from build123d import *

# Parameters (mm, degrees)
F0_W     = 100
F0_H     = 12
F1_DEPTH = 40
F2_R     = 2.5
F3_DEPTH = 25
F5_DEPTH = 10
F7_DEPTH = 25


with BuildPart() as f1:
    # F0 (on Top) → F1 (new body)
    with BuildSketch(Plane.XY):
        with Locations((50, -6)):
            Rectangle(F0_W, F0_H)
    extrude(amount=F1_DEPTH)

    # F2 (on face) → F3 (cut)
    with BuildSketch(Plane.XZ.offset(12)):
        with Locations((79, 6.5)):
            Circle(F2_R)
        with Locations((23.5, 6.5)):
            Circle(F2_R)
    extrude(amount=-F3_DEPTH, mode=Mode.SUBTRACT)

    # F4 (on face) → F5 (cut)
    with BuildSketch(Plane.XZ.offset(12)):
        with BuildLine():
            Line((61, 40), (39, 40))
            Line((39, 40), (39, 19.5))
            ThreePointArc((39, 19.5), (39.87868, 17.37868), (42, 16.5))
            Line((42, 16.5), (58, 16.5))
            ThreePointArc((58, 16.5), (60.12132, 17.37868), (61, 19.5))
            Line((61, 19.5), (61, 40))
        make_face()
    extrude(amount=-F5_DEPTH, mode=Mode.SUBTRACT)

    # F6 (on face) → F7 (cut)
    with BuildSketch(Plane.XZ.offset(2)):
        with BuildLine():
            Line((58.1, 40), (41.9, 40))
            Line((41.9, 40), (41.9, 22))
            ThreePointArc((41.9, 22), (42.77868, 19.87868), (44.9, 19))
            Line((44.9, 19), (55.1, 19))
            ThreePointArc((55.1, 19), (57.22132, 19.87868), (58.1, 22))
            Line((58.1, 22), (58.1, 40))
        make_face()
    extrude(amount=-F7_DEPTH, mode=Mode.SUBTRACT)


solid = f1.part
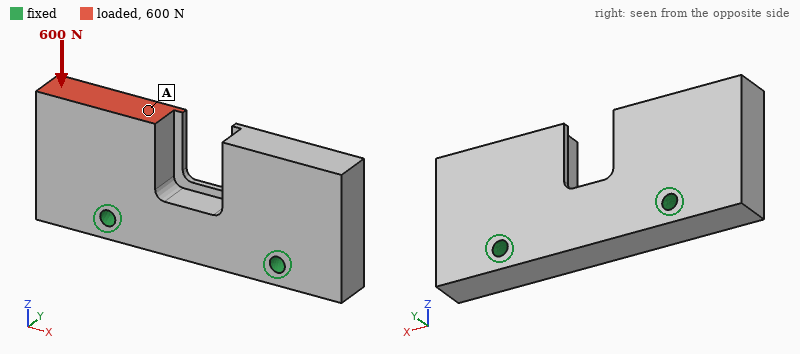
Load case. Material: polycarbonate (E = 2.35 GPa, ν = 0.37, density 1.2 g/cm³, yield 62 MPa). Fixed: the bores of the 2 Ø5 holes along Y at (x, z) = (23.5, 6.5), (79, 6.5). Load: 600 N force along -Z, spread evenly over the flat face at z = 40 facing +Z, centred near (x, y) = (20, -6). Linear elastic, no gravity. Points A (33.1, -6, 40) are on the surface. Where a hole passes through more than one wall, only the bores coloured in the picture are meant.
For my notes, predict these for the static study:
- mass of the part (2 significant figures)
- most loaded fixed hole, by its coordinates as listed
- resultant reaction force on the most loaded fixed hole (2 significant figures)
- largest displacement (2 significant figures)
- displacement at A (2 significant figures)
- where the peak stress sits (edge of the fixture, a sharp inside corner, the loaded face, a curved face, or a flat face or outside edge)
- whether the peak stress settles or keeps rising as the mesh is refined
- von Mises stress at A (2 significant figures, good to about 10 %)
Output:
50 g
(23.5, 6.5)
620 N
97 µm
55 µm
edge of the fixture
keeps rising
1.3 MPa
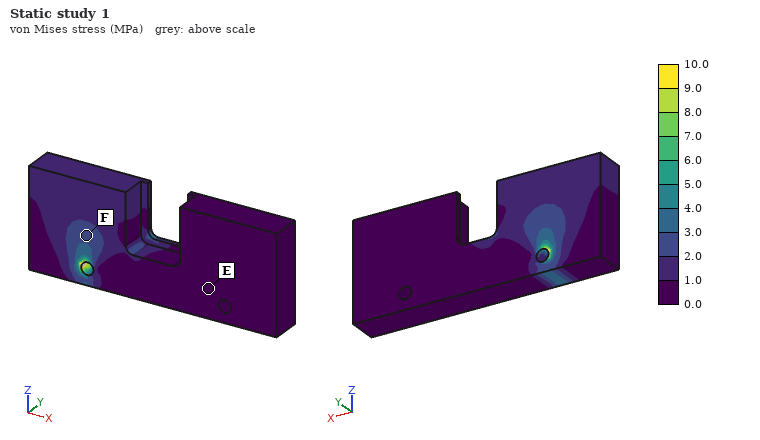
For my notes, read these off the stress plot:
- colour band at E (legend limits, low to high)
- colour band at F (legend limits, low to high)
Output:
0.0 to 1.0 MPa
2.0 to 3.0 MPa
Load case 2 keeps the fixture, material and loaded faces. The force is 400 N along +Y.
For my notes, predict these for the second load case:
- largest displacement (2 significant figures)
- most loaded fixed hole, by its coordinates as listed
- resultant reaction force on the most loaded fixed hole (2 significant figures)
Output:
0.66 mm
(23.5, 6.5)
420 N
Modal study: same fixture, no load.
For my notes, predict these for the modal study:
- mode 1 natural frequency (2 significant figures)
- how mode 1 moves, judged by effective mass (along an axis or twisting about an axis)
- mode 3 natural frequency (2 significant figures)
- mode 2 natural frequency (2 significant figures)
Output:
1700 Hz
along Y
1900 Hz
1800 Hz
